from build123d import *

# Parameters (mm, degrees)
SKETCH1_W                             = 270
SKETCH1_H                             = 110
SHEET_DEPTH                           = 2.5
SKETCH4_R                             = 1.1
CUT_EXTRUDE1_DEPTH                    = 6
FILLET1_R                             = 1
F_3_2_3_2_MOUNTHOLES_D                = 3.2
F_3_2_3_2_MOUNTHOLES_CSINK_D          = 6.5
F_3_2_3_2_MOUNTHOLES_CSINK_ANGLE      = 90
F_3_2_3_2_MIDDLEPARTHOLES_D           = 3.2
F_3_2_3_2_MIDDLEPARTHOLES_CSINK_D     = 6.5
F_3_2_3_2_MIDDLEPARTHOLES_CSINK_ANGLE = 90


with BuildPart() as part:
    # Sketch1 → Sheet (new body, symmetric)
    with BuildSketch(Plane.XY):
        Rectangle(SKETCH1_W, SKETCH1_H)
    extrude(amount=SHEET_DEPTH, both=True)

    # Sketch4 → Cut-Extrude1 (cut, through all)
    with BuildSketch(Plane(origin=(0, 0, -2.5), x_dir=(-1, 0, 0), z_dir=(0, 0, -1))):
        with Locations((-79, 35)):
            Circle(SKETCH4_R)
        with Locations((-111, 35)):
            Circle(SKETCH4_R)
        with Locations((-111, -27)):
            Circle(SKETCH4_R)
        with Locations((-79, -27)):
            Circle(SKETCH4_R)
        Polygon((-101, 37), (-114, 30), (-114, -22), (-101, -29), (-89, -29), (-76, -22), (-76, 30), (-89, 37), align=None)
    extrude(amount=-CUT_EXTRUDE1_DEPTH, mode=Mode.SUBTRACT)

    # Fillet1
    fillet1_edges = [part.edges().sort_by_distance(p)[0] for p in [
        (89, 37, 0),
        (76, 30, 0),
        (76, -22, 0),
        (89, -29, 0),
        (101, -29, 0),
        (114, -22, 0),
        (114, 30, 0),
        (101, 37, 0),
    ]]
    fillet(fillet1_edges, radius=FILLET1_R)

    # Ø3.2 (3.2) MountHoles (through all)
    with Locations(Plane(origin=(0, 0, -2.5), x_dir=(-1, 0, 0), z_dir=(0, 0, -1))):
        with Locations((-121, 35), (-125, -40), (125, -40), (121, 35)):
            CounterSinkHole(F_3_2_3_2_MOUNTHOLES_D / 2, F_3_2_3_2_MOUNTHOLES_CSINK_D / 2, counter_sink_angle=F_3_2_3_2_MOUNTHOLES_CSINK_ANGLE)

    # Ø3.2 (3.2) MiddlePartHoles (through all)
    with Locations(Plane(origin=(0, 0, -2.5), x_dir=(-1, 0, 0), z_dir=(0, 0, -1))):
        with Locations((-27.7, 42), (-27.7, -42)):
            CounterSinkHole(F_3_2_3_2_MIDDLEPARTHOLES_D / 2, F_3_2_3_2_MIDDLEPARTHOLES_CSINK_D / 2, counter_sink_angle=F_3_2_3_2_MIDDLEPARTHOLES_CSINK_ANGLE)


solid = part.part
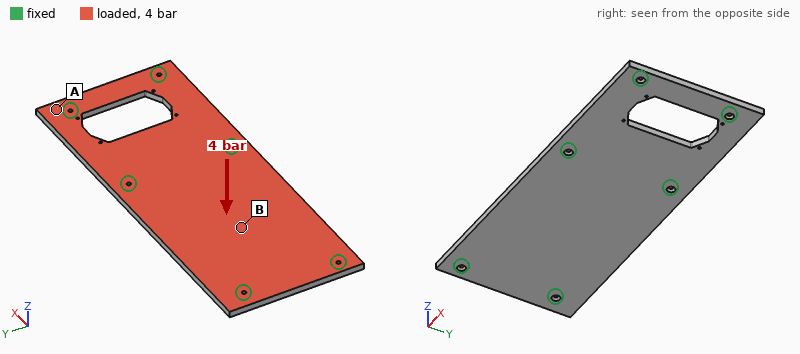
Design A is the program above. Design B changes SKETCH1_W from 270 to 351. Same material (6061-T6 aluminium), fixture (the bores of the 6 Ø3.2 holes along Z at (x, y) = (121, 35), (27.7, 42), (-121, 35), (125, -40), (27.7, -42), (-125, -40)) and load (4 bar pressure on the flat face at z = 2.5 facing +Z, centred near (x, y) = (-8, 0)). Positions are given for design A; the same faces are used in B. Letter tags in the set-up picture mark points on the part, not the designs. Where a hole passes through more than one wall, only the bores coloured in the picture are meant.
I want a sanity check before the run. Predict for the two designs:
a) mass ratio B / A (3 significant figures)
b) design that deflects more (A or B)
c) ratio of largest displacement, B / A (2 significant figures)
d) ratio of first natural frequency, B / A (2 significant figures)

1.33
A
0.91
0.94
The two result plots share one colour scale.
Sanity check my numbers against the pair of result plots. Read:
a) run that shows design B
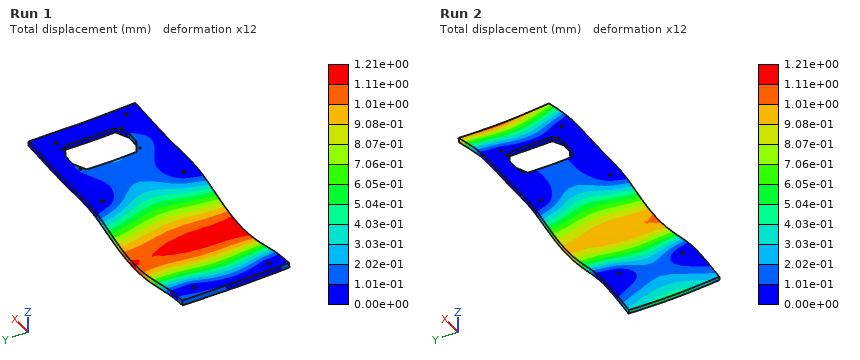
Run 2
